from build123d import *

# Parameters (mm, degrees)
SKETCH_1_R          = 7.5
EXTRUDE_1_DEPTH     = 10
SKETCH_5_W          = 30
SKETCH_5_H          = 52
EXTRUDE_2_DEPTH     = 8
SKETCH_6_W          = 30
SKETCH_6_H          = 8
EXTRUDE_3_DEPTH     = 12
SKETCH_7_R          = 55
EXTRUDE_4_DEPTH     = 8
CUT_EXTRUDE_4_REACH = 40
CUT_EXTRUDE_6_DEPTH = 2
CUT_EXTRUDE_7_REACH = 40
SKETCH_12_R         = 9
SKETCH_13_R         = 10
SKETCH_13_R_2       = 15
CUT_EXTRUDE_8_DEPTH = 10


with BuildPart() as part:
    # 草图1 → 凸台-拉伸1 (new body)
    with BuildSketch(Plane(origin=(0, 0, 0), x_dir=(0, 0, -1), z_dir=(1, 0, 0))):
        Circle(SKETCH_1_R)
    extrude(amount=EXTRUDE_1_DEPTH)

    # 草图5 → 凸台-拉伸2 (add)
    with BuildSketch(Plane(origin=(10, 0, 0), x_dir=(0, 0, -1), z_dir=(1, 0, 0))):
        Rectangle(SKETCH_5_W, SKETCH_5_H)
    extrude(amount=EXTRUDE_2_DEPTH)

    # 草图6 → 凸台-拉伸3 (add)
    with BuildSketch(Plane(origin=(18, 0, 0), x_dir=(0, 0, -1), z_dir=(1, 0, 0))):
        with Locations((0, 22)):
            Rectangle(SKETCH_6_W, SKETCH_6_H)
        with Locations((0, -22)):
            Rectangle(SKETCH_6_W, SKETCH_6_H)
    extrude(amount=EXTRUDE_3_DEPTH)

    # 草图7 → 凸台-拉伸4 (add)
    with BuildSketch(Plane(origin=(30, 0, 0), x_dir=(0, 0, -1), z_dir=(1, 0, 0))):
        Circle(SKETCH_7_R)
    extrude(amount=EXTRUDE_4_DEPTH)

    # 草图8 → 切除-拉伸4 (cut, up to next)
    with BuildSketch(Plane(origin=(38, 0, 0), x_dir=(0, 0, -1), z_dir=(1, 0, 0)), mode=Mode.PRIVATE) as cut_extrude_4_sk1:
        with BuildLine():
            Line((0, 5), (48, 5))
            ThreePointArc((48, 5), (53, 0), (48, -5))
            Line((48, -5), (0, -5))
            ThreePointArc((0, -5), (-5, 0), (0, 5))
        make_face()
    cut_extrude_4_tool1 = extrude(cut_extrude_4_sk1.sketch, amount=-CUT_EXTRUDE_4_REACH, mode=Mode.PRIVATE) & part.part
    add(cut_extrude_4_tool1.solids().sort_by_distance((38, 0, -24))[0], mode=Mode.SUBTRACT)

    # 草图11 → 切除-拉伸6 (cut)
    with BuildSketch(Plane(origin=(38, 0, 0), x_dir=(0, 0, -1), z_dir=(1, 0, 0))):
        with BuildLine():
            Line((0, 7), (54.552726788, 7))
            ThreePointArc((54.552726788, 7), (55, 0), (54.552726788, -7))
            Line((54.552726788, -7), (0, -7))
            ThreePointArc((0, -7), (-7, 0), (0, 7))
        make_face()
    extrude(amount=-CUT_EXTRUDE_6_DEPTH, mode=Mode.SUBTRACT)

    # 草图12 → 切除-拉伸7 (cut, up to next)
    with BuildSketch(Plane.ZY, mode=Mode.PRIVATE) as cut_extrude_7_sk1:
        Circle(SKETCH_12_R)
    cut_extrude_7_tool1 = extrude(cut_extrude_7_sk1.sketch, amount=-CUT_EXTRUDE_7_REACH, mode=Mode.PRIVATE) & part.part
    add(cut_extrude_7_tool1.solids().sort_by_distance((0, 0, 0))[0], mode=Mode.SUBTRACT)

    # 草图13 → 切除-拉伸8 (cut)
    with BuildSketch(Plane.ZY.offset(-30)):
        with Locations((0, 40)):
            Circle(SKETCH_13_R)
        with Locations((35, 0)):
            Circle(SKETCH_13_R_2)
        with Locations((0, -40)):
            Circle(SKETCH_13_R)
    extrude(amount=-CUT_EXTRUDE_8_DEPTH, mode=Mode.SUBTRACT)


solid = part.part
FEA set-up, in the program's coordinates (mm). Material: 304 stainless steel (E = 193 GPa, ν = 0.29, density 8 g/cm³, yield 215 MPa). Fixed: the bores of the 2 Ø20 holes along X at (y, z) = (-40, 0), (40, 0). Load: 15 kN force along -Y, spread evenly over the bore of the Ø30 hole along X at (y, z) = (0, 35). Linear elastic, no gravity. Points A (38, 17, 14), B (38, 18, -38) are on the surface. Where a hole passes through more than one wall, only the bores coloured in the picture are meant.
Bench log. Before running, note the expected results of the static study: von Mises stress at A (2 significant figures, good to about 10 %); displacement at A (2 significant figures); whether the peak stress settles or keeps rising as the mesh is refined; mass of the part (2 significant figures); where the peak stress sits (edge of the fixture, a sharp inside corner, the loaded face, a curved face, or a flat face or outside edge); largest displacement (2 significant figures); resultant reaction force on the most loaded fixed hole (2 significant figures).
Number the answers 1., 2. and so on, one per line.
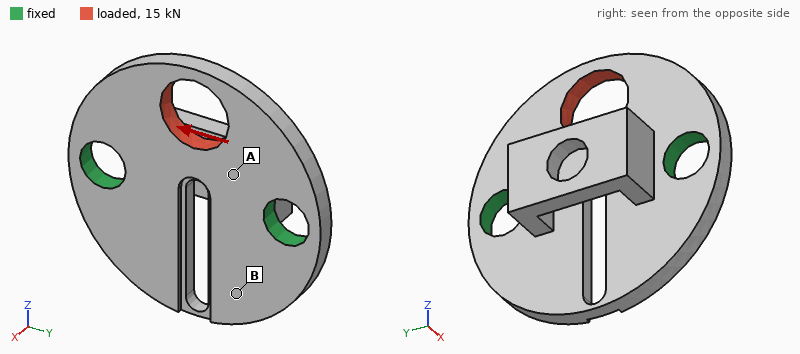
1. 29 MPa
2. 4.6 µm
3. keeps rising
4. 610 g
5. a sharp inside corner
6. 26 µm
7. 8.7 kN
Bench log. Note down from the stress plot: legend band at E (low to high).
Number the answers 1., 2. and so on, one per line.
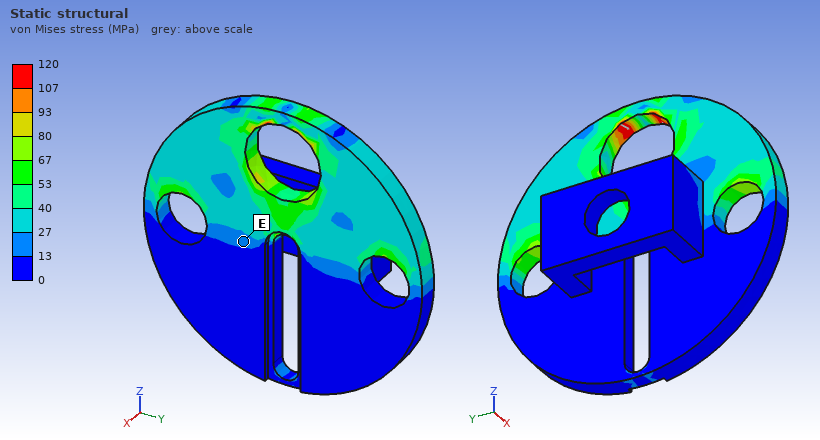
1. 13 to 27 MPa
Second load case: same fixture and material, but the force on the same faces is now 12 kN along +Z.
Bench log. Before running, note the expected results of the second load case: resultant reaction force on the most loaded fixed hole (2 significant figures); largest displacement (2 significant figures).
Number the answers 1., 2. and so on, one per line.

1. 6.6 kN
2. 16 µm
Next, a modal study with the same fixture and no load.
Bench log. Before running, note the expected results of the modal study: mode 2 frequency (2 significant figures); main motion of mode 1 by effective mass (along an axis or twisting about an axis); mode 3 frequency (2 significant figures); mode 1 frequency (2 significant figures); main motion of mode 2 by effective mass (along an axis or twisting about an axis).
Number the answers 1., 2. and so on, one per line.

1. 3800 Hz
2. twisting about Y
3. 6000 Hz
4. 3100 Hz
5. along X
